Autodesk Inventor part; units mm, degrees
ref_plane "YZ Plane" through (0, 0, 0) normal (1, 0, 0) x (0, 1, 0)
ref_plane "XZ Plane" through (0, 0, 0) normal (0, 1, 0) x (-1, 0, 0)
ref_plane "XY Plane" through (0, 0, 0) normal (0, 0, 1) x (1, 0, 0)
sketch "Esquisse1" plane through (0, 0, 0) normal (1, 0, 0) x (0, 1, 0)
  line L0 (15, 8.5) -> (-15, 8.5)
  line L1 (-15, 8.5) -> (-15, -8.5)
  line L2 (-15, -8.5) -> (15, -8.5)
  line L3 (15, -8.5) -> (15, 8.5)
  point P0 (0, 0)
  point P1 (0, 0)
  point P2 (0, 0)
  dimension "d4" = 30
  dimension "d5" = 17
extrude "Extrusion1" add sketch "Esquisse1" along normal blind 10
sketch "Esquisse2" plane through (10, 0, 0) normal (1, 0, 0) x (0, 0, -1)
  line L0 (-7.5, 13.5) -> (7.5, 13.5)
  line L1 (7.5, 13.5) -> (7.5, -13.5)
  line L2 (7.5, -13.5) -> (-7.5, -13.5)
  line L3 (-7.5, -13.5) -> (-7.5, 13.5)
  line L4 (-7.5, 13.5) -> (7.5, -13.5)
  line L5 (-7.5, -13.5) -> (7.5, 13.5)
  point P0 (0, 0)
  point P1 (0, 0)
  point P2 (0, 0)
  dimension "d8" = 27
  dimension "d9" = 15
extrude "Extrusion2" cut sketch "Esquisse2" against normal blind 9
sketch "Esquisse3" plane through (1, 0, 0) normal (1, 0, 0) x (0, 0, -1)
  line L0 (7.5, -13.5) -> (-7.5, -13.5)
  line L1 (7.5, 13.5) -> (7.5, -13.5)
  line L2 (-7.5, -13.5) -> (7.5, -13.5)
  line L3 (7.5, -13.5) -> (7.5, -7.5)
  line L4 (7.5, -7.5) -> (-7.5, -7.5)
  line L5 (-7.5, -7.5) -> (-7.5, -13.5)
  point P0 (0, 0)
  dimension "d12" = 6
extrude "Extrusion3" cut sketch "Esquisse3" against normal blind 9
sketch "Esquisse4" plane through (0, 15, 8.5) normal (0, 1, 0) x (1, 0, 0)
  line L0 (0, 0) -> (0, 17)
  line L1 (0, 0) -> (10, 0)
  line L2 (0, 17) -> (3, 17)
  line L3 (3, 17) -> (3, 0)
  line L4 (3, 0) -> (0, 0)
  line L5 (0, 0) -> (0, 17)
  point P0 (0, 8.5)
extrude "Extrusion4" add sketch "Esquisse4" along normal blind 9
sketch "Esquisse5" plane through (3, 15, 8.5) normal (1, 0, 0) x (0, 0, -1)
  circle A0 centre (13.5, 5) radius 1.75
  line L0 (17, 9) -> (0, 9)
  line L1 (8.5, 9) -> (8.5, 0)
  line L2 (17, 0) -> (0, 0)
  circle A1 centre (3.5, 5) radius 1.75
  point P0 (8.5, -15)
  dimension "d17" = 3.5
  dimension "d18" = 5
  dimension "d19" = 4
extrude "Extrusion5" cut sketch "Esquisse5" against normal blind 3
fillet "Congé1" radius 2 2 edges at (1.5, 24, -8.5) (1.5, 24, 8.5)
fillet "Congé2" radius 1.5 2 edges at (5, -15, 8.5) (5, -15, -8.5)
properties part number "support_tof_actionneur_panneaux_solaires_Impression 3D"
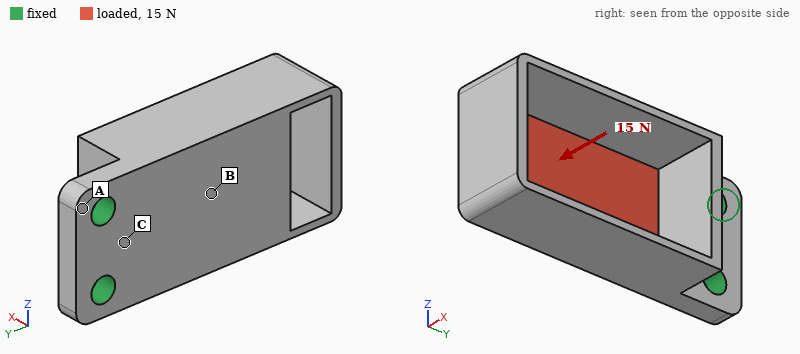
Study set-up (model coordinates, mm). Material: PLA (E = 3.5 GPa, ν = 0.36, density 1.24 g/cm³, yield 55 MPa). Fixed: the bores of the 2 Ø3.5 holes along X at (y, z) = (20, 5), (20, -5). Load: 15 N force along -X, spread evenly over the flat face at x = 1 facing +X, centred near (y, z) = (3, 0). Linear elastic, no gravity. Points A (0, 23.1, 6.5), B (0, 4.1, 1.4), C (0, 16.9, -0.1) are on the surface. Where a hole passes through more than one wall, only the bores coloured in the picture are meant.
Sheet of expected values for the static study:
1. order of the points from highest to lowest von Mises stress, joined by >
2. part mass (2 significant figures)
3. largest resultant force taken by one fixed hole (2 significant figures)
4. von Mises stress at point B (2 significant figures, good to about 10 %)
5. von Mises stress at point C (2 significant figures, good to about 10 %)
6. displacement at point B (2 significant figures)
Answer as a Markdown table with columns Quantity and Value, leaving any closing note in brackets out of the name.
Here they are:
| Quantity | Value |
|---|---|
| order of the points from highest to lowest von Mises stress, joined by > | C > B > A |
| part mass | 2.2 g |
| largest resultant force taken by one fixed hole | 8.7 N |
| von Mises stress at point B | 2.9 MPa |
| von Mises stress at point C | 5.0 MPa |
| displacement at point B | 0.19 mm |
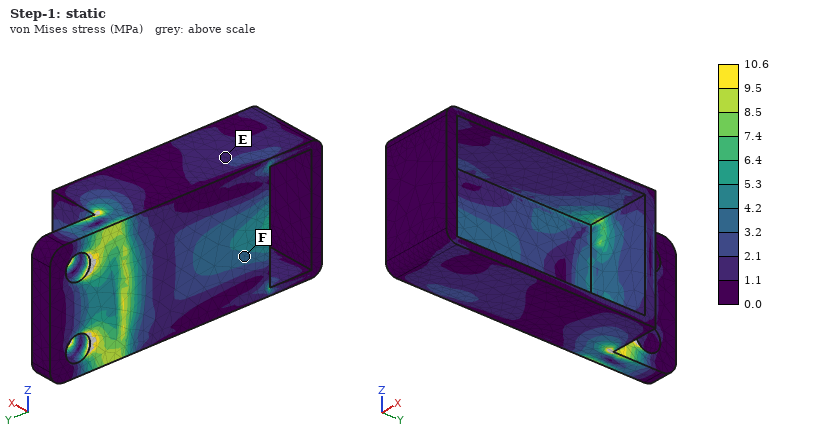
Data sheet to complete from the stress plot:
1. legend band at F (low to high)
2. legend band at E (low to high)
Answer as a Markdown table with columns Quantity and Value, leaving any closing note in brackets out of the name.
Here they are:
| Quantity | Value |
|---|---|
| legend band at F | 3.2 to 4.2 MPa |
| legend band at E | 1.1 to 2.1 MPa |
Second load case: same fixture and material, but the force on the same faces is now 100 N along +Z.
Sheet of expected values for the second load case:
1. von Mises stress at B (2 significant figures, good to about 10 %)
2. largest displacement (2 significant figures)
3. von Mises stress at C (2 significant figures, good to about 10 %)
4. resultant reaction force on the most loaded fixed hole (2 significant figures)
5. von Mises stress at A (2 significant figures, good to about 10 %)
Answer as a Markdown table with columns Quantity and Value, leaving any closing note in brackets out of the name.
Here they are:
| Quantity | Value |
|---|---|
| von Mises stress at B | 5.5 MPa |
| largest displacement | 0.49 mm |
| von Mises stress at C | 3.7 MPa |
| resultant reaction force on the most loaded fixed hole | 140 N |
| von Mises stress at A | 1.3 MPa |
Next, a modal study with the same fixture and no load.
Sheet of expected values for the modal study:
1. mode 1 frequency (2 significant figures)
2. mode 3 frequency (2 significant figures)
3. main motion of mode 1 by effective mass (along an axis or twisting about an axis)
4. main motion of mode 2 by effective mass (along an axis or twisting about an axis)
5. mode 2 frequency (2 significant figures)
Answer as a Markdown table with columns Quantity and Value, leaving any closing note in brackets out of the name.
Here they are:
| Quantity | Value |
|---|---|
| mode 1 frequency | 780 Hz |
| mode 3 frequency | 2100 Hz |
| main motion of mode 1 by effective mass | along X |
| main motion of mode 2 by effective mass | along Z |
| mode 2 frequency | 1000 Hz |
